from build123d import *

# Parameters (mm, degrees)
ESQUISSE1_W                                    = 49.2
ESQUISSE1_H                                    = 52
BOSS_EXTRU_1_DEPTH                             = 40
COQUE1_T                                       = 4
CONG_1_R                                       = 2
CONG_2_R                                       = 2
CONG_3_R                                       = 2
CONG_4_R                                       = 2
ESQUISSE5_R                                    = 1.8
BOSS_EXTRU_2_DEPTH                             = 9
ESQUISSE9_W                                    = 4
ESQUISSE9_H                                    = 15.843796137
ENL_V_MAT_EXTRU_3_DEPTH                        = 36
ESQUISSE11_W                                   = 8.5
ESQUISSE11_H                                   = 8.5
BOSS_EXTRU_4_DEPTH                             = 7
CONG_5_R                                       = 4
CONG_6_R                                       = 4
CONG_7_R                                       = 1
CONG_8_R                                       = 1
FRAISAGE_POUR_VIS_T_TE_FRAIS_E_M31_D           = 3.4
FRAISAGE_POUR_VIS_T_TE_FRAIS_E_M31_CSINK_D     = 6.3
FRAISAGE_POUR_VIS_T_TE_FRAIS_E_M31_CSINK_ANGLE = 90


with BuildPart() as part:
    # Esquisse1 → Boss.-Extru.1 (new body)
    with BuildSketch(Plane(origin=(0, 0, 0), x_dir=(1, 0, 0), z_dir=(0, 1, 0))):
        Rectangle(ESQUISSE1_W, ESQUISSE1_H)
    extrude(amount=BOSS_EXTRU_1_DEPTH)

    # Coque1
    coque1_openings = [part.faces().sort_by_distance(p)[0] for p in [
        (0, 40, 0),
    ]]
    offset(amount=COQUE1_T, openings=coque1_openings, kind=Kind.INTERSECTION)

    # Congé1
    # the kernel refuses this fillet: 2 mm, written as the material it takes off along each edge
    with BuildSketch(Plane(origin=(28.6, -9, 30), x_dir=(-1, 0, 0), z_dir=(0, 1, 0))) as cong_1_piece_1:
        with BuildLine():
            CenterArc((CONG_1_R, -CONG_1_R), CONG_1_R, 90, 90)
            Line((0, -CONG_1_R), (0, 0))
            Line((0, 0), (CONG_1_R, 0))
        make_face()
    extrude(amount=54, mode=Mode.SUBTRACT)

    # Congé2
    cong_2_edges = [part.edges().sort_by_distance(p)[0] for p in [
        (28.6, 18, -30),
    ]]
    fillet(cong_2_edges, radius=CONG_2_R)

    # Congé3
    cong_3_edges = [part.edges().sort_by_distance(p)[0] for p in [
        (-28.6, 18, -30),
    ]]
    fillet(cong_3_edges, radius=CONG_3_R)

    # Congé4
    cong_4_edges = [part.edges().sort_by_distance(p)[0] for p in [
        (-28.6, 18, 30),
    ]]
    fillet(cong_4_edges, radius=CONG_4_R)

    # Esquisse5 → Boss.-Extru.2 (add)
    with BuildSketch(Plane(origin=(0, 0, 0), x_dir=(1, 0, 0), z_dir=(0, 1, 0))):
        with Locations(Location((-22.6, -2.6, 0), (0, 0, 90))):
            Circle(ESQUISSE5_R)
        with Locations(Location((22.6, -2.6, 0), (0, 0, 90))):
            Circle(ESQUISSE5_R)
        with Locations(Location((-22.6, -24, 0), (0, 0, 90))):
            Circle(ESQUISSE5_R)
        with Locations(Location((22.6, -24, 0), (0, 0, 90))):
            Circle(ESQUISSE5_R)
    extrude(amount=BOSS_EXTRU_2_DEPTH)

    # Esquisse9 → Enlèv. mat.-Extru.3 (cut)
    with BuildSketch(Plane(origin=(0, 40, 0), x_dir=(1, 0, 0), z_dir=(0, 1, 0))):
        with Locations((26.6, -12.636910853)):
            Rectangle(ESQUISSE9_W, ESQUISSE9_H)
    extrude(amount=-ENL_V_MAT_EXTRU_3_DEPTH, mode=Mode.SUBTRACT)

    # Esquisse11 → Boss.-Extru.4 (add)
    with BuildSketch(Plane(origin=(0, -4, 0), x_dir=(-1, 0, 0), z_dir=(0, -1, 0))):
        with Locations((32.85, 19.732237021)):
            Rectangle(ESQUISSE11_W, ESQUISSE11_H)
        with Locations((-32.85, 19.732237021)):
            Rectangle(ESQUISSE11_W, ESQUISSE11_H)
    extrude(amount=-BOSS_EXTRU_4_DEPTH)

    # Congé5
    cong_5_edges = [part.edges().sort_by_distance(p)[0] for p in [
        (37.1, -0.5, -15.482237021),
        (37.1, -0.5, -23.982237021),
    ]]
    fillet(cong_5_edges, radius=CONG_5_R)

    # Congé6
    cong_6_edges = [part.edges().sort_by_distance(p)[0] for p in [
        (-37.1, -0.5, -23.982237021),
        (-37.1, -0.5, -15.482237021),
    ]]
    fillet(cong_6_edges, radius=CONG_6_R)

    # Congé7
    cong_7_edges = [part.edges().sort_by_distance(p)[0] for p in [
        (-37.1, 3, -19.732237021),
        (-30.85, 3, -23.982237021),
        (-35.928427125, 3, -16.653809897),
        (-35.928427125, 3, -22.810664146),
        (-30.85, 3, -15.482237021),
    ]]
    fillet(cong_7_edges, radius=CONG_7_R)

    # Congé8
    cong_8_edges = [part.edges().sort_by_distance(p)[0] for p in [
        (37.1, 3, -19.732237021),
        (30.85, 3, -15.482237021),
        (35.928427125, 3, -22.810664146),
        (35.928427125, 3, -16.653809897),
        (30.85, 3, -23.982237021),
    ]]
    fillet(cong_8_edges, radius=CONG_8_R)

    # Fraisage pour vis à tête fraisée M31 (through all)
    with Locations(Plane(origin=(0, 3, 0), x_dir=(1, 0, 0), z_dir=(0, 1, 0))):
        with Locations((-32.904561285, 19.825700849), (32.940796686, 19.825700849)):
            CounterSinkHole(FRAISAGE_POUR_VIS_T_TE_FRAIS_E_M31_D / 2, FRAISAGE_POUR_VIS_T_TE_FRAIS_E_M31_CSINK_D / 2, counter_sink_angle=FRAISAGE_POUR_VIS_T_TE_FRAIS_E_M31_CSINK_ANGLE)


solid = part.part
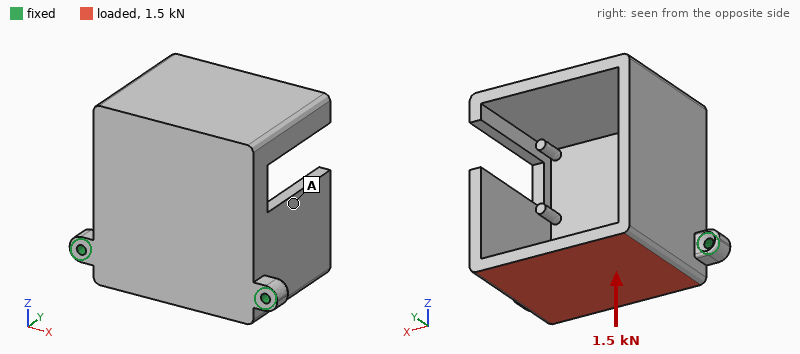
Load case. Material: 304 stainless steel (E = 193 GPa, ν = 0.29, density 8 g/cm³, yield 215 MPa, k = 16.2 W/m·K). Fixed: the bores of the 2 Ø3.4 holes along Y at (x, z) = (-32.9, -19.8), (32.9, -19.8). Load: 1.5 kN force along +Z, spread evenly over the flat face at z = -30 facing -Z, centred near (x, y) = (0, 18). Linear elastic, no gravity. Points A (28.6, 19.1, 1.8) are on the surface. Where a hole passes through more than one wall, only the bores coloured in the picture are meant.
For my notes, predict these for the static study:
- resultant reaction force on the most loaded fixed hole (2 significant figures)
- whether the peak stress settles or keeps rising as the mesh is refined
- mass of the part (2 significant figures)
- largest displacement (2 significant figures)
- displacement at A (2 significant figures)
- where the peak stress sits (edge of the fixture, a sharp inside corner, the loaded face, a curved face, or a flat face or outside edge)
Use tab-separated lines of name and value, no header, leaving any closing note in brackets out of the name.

resultant reaction force on the most loaded fixed hole	750 N
whether the peak stress settles or keeps rising as the mesh is refined	keeps rising
mass of the part	380 g
largest displacement	0.16 mm
displacement at A	0.071 mm
where the peak stress sits	edge of the fixture
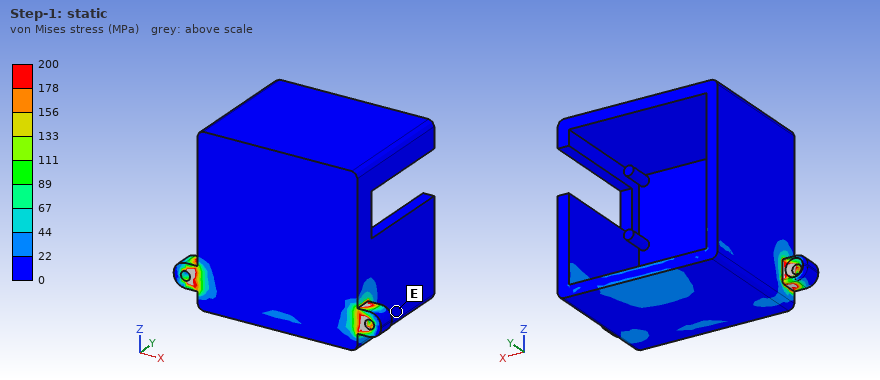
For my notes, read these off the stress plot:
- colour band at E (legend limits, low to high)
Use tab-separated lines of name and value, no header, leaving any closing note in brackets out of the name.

colour band at E	0 to 22 MPa
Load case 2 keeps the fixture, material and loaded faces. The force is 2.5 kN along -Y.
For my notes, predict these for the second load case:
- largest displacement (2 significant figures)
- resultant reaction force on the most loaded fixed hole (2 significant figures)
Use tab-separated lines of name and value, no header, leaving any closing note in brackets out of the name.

largest displacement	0.14 mm
resultant reaction force on the most loaded fixed hole	1.3 kN
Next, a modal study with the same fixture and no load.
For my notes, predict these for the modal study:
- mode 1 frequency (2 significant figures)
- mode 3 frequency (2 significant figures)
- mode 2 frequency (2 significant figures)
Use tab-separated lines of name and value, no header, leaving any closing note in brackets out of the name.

mode 1 frequency	770 Hz
mode 3 frequency	2500 Hz
mode 2 frequency	1600 Hz
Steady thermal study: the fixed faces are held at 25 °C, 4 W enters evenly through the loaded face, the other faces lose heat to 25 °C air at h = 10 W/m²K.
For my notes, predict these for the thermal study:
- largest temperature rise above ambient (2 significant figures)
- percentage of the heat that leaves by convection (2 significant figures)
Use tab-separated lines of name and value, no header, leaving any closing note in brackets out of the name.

largest temperature rise above ambient	21 K
percentage of the heat that leaves by convection	46 %
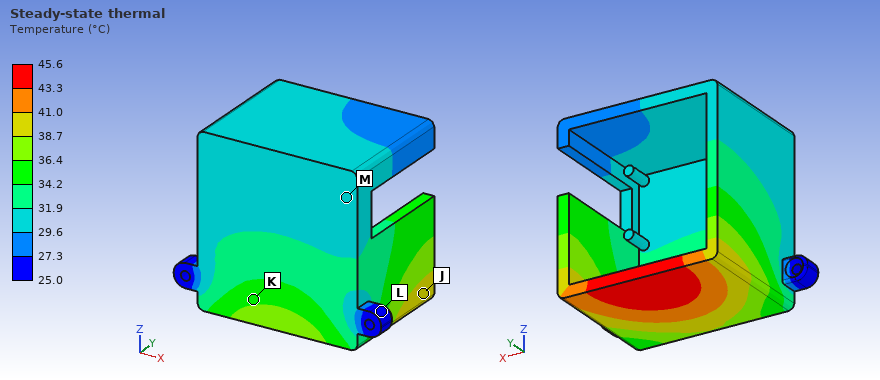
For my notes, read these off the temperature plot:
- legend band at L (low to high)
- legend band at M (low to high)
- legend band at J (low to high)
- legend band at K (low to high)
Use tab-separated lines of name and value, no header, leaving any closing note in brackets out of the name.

legend band at L	25.0 to 27.3 °C
legend band at M	29.6 to 31.9 °C
legend band at J	38.7 to 41.0 °C
legend band at K	34.2 to 36.4 °C
